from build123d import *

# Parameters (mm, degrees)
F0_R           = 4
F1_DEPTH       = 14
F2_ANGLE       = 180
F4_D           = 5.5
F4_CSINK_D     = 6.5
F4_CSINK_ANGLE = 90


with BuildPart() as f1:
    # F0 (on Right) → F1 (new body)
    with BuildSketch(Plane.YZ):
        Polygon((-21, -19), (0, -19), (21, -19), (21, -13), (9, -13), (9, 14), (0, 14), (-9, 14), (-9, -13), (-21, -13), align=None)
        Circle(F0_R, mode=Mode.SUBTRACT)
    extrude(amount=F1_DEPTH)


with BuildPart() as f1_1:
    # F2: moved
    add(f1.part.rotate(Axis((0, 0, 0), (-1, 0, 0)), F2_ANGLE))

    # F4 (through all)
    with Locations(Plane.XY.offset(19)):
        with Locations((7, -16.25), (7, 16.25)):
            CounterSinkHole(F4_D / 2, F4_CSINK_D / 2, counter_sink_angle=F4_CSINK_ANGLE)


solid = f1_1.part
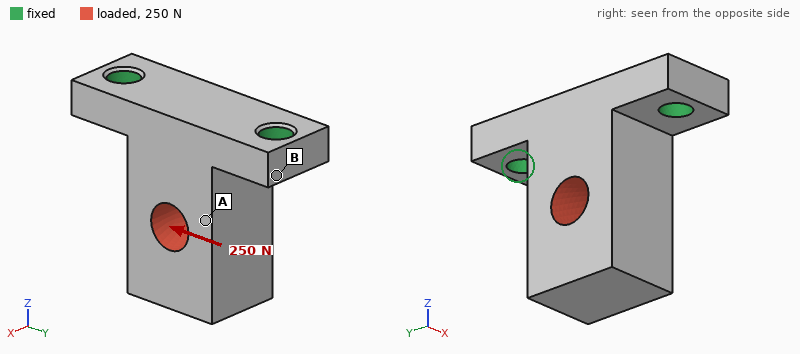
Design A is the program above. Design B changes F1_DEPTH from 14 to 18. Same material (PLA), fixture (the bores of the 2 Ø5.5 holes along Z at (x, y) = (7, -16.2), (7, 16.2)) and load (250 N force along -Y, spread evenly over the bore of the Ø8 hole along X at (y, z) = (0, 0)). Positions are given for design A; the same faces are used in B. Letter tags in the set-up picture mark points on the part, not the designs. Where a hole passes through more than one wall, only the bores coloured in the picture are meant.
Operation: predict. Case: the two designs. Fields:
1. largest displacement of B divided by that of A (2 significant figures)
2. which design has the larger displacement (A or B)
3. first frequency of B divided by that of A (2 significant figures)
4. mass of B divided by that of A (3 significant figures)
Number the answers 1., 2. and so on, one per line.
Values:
1. 0.85
2. A
3. 1.0
4. 1.29
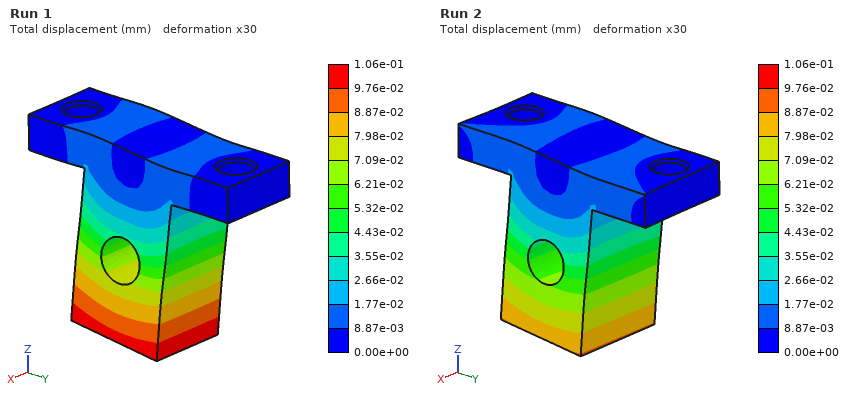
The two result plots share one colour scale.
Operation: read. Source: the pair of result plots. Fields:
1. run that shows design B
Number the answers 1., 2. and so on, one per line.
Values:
1. Run 2
